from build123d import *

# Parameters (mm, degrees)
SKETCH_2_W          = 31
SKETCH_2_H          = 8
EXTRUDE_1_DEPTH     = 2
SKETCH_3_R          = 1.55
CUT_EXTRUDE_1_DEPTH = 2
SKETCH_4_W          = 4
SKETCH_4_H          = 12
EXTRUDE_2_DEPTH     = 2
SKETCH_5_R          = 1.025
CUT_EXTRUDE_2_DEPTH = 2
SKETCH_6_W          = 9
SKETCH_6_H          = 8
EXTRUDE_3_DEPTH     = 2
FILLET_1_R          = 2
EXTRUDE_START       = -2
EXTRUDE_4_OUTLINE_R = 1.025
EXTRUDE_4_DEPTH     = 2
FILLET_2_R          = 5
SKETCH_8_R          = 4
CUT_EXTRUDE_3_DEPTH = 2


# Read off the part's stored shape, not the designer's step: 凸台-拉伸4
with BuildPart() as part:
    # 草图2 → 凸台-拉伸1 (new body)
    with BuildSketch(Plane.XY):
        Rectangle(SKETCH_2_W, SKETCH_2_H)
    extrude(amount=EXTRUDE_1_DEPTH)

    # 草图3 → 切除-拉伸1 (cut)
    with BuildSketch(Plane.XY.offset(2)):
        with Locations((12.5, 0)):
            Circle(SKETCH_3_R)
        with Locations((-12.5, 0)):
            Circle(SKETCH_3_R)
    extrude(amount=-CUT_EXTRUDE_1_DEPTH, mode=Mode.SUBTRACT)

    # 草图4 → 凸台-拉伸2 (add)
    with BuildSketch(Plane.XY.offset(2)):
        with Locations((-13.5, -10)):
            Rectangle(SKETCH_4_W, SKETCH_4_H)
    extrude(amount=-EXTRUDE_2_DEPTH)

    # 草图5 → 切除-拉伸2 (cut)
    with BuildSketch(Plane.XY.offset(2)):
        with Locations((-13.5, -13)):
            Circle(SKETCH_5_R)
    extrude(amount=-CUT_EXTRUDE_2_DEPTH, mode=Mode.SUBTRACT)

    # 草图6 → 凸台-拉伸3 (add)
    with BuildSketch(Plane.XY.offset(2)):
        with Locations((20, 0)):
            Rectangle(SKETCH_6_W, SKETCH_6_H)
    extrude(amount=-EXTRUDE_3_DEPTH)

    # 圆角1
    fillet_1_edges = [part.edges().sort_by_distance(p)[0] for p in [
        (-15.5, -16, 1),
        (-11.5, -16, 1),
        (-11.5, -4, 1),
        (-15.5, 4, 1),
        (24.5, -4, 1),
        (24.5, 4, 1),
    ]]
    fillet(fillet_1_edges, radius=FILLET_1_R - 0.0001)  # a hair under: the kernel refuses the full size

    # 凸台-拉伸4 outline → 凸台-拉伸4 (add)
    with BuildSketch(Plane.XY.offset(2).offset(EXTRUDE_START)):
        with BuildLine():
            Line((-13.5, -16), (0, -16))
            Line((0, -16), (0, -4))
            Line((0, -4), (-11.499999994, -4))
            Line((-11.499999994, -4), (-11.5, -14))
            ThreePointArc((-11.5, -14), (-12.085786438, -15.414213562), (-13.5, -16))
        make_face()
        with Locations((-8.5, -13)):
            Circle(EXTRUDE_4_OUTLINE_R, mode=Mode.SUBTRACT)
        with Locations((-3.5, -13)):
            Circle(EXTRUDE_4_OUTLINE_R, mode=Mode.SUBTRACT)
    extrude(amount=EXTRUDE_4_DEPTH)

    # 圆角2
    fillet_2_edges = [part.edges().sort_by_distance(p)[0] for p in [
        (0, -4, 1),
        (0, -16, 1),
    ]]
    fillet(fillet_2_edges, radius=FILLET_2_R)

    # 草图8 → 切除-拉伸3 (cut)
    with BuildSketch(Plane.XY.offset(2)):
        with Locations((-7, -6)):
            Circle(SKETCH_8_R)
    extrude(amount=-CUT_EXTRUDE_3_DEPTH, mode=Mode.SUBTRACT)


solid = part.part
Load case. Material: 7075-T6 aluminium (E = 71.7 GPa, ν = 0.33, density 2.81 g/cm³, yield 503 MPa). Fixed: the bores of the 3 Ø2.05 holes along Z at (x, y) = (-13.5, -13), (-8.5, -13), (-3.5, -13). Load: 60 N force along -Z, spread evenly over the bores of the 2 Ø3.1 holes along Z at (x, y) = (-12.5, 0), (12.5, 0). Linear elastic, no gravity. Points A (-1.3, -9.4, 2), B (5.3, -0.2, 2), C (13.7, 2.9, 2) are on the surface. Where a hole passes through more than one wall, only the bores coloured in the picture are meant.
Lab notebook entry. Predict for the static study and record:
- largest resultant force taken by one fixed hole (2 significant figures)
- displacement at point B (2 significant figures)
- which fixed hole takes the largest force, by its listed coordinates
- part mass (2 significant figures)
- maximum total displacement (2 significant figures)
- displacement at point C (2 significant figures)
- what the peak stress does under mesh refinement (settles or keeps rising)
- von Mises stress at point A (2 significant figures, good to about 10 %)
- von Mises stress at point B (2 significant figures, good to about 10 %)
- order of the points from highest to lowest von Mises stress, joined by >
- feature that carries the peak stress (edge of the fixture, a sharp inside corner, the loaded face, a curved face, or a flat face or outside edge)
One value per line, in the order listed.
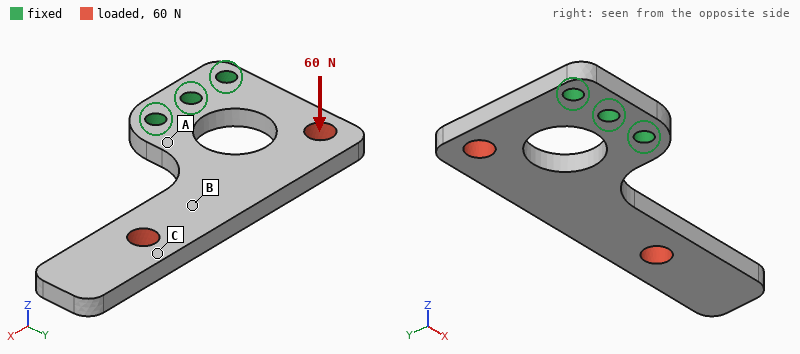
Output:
67 N
0.18 mm
(-3.5, -13)
2.4 g
0.50 mm
0.34 mm
keeps rising
140 MPa
40 MPa
A > B > C
edge of the fixture
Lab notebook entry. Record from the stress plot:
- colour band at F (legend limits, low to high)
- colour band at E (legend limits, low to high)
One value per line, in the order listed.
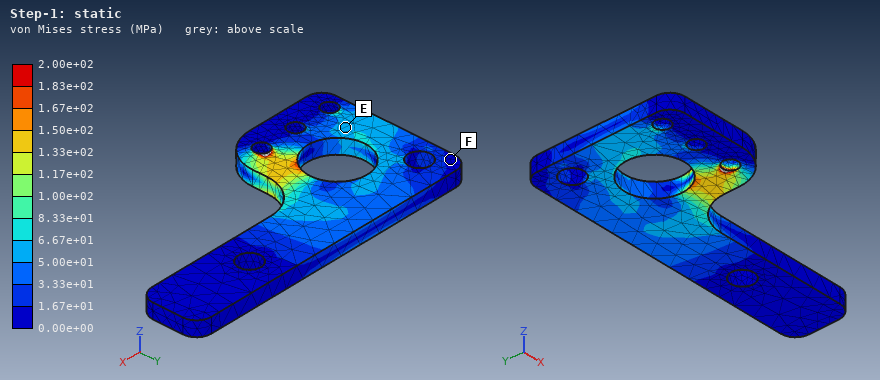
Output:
0.00e+00 to 1.67e+01 MPa
5.00e+01 to 6.67e+01 MPa
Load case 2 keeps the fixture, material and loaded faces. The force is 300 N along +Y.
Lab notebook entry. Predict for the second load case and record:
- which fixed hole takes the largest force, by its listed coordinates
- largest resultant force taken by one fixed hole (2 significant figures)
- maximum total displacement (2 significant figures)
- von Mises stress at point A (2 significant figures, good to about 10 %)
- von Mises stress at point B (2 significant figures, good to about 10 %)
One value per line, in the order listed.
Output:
(-3.5, -13)
330 N
92 µm
49 MPa
23 MPa
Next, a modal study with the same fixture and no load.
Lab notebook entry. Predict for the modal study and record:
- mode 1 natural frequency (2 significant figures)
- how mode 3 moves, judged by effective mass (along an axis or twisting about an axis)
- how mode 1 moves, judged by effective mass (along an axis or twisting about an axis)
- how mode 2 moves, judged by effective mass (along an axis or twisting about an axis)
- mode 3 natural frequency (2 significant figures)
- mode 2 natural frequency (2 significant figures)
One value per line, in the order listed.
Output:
1500 Hz
along Y
along Z
along Z
7000 Hz
4300 Hz
